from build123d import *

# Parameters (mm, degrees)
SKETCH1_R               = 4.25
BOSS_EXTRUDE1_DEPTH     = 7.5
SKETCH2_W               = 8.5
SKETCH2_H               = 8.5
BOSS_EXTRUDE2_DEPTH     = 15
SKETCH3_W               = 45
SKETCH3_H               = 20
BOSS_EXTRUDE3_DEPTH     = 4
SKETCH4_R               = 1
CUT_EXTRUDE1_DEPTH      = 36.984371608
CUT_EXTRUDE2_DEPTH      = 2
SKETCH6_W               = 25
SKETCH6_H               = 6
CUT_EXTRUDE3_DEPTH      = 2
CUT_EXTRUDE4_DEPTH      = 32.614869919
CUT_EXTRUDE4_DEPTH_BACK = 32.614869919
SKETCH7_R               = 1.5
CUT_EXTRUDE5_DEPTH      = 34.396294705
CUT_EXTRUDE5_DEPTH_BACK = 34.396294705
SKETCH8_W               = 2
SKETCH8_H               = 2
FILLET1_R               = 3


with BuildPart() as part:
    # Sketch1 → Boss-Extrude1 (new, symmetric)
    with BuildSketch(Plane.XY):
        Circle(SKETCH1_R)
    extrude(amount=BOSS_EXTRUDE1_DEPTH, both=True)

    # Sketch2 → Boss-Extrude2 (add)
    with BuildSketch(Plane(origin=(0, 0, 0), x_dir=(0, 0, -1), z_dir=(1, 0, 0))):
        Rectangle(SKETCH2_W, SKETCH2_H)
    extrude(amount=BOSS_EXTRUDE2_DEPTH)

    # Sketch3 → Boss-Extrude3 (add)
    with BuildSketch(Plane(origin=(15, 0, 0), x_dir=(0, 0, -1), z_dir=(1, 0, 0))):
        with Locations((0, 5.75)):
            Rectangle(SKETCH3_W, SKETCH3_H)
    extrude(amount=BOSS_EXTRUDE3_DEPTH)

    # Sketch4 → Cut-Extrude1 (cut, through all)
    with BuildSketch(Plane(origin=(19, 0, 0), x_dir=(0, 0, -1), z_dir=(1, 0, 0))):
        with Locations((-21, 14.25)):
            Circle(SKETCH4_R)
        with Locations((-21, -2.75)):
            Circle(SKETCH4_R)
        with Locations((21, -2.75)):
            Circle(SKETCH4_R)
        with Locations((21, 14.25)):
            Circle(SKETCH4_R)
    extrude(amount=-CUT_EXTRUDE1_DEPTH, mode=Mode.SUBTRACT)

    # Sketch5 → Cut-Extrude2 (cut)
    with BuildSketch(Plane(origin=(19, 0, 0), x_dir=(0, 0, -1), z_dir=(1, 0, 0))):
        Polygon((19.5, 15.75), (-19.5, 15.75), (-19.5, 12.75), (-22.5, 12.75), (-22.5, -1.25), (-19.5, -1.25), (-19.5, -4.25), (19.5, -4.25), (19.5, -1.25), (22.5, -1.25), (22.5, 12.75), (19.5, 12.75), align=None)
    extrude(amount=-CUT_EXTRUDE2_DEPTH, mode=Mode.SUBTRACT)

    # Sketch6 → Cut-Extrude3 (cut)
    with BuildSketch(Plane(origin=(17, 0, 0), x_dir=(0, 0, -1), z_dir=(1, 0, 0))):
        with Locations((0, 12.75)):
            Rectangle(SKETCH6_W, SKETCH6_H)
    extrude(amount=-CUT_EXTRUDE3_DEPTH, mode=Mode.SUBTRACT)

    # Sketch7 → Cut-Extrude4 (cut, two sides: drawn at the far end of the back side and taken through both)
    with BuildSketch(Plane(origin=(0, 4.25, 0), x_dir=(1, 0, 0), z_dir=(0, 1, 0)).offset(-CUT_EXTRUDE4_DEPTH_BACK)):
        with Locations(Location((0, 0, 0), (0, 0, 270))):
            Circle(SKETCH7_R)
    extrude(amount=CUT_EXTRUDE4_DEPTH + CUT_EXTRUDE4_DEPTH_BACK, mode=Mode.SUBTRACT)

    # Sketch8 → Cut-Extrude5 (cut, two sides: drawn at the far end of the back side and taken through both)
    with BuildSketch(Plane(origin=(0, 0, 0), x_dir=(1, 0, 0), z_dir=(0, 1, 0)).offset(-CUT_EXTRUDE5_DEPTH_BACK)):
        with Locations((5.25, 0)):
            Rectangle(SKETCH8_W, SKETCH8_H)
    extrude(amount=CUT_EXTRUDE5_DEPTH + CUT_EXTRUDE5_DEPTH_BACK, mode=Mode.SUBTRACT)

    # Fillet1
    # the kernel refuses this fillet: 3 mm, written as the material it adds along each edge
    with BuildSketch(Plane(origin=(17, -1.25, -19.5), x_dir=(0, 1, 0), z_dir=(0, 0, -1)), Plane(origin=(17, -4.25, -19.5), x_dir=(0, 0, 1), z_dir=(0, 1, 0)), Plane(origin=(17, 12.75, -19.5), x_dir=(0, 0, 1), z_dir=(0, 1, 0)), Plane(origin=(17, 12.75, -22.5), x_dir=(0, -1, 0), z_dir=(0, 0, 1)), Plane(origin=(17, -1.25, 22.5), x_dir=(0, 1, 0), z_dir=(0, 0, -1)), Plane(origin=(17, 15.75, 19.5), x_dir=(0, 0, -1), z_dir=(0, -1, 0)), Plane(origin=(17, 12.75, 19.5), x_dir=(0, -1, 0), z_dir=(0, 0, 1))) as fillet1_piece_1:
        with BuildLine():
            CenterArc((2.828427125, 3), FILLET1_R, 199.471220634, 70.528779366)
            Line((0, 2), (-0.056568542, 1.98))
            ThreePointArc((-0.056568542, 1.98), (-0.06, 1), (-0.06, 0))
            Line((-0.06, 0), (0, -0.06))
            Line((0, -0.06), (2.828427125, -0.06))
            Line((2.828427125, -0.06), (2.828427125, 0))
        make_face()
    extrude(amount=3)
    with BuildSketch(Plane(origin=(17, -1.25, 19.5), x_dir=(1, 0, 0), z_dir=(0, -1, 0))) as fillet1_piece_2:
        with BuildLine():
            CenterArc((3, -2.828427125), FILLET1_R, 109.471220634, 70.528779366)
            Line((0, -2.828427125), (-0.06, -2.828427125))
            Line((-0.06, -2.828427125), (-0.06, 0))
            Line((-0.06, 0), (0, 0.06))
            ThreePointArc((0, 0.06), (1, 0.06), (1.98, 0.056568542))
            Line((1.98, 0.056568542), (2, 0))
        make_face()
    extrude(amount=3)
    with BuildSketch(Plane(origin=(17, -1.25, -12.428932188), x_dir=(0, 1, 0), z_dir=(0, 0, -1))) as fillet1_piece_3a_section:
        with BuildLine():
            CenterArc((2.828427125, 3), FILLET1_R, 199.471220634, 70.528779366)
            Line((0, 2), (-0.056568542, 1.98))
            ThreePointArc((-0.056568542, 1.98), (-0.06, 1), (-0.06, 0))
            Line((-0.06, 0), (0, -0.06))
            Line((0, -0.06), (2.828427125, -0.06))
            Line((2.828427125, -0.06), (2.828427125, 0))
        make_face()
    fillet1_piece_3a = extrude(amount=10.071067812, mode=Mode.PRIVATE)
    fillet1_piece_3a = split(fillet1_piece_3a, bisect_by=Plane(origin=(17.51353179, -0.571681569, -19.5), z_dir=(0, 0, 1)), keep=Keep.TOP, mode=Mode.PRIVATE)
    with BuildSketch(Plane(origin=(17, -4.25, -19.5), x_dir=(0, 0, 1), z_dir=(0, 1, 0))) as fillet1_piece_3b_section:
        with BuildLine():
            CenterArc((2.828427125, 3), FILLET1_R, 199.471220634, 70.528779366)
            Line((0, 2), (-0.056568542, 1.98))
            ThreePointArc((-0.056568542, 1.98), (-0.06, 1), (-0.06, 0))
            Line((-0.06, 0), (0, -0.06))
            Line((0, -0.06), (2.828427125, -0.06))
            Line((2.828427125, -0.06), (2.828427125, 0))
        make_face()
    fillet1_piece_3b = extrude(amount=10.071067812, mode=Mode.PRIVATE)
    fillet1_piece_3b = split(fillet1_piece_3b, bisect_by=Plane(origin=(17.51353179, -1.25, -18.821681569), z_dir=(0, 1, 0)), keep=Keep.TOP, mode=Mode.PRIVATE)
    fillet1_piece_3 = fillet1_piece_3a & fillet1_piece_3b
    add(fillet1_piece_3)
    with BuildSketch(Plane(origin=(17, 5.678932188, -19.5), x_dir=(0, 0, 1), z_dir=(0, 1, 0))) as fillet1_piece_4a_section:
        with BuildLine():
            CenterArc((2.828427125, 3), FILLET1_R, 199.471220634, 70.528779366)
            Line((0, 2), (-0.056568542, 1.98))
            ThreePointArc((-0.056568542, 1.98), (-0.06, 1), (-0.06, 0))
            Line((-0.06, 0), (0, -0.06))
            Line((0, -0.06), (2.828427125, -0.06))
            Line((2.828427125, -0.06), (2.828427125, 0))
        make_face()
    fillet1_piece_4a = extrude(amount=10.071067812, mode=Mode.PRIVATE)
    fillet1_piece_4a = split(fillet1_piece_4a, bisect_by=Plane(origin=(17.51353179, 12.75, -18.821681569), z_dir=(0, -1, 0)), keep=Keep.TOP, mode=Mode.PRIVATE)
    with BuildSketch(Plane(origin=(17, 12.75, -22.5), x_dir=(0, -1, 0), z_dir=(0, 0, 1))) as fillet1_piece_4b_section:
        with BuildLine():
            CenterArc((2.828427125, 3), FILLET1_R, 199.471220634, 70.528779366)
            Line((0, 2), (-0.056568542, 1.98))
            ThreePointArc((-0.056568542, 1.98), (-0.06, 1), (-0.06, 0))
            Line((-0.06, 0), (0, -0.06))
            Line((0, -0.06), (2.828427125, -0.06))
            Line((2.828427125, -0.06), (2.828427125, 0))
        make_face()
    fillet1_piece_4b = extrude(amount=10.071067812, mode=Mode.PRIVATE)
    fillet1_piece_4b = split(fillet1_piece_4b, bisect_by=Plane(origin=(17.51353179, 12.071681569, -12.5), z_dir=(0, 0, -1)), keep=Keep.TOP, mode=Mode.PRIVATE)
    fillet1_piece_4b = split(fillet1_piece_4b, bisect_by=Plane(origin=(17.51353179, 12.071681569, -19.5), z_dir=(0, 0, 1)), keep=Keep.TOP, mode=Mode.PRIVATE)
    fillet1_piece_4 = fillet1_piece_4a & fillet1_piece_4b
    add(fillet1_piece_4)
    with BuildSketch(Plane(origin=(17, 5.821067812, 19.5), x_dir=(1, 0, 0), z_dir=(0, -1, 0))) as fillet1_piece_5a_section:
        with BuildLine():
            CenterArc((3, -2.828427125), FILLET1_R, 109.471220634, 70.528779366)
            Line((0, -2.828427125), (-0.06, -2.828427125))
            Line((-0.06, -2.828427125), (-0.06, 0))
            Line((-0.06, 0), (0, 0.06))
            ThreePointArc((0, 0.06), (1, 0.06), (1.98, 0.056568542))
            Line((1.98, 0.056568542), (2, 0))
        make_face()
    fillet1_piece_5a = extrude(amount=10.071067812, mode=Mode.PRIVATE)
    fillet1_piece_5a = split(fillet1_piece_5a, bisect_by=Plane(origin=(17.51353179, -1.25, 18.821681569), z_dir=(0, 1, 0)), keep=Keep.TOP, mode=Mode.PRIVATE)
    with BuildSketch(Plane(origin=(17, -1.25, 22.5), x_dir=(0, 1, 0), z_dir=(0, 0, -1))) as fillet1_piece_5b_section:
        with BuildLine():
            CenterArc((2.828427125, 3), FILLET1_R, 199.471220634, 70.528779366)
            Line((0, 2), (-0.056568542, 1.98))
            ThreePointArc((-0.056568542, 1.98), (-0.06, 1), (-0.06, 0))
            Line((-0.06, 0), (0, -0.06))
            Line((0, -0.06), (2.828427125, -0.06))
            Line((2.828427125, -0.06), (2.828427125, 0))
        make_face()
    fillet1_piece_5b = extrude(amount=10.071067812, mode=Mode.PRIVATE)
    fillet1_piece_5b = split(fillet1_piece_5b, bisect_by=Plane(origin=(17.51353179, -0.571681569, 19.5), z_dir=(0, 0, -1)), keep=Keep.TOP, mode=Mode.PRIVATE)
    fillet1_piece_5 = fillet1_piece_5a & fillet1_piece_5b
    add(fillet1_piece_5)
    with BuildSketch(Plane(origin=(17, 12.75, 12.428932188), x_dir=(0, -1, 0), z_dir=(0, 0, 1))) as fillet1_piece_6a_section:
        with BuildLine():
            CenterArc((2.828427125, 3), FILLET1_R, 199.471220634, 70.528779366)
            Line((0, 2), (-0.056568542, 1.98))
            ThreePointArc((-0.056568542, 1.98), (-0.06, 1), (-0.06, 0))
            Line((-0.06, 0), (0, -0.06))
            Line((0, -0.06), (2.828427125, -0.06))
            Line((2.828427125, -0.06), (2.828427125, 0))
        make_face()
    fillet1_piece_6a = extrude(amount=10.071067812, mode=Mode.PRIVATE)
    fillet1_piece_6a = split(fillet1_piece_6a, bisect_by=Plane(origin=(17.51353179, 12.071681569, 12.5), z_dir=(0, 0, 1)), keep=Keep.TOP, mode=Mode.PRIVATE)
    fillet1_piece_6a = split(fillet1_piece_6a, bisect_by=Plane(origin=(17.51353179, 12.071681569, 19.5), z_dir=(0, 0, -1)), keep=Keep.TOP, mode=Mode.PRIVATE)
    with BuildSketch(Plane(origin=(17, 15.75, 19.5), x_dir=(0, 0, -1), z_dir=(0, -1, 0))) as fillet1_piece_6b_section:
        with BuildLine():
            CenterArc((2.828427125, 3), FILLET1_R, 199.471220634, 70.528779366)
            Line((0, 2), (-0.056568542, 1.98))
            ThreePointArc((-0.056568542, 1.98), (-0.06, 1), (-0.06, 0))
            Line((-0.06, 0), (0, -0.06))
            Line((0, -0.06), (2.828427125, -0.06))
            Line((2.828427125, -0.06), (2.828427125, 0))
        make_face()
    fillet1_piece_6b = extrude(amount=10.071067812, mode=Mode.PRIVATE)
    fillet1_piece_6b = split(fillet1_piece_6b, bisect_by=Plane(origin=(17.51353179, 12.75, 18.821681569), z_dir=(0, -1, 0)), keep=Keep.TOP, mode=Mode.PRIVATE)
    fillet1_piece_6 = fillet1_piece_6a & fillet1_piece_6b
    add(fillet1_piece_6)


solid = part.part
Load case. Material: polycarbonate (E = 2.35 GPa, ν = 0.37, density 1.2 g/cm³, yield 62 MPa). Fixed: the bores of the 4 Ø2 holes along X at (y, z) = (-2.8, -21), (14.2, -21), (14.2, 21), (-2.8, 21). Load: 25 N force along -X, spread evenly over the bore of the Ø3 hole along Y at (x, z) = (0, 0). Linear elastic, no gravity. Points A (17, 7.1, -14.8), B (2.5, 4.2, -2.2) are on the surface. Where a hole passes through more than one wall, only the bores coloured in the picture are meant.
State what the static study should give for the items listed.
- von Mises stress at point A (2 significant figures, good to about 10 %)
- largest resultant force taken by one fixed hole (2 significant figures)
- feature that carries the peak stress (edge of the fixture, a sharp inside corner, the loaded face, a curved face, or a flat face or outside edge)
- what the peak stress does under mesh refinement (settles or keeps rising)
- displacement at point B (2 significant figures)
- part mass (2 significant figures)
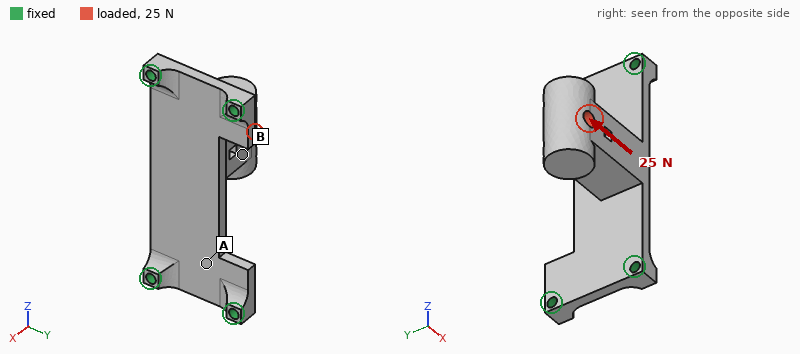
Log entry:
3.6 MPa
15 N
edge of the fixture
keeps rising
0.25 mm
3.8 g
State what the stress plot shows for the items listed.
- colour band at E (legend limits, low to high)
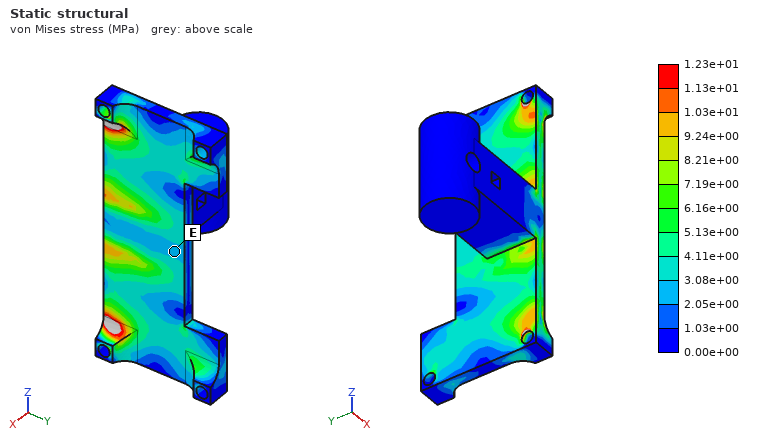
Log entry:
2.05e+00 to 3.08e+00 MPa
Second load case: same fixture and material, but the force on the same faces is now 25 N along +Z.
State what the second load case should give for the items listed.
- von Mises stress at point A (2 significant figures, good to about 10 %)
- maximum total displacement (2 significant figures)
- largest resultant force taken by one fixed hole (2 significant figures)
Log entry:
1.9 MPa
0.56 mm
14 N
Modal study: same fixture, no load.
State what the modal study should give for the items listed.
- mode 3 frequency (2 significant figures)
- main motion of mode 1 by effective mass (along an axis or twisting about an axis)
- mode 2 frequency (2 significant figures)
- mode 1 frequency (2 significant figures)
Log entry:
1100 Hz
along Y
1100 Hz
650 Hz
